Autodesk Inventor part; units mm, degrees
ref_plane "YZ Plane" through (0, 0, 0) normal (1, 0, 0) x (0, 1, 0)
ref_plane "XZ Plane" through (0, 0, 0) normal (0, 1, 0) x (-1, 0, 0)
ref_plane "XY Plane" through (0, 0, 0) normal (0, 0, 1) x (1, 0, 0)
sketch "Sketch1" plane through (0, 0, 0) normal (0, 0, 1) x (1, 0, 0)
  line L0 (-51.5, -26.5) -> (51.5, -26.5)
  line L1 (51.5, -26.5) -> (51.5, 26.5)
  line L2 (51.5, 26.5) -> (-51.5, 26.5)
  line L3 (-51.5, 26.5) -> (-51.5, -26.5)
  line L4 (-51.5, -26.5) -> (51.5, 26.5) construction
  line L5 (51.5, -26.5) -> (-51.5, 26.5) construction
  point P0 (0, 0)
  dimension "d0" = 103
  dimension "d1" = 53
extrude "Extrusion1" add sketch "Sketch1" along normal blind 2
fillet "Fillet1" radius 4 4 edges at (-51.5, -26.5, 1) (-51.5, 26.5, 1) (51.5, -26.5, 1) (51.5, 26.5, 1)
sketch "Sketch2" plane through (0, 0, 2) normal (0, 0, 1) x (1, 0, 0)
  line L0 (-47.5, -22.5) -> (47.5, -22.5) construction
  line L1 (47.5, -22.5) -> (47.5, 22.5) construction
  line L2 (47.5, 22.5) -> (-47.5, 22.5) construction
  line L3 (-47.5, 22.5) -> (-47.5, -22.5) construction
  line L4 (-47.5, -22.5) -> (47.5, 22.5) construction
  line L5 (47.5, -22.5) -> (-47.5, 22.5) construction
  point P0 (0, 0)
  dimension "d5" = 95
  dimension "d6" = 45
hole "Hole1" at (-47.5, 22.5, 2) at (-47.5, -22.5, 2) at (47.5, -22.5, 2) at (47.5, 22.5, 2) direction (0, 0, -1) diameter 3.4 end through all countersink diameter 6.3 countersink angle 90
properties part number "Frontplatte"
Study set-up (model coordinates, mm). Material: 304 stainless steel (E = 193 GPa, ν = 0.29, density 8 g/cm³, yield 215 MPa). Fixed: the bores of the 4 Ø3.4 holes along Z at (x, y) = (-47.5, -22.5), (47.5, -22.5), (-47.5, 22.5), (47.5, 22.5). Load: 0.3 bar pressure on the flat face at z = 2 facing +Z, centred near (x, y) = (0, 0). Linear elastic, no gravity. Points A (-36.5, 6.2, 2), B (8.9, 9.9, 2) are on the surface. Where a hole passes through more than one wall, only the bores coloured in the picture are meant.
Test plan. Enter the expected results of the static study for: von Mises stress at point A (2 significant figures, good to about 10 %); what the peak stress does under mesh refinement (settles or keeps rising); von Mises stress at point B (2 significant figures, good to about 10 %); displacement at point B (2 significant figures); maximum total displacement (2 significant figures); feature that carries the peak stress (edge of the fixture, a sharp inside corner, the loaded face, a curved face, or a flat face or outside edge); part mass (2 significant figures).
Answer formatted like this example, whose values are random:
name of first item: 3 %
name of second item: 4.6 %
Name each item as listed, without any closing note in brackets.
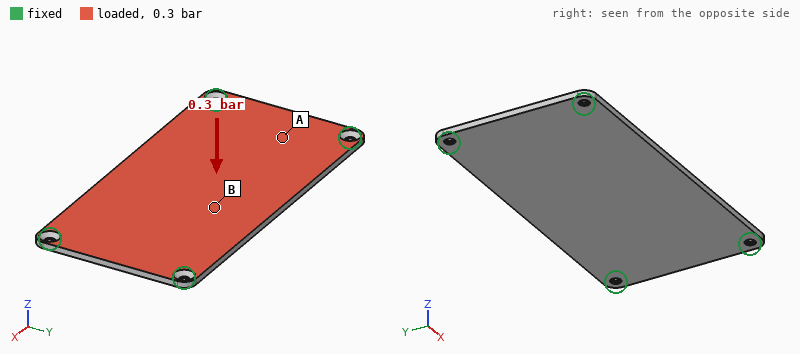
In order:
von Mises stress at point A: 9.1 MPa
what the peak stress does under mesh refinement: keeps rising
von Mises stress at point B: 22 MPa
displacement at point B: 80 µm
maximum total displacement: 87 µm
feature that carries the peak stress: edge of the fixture
part mass: 86 g
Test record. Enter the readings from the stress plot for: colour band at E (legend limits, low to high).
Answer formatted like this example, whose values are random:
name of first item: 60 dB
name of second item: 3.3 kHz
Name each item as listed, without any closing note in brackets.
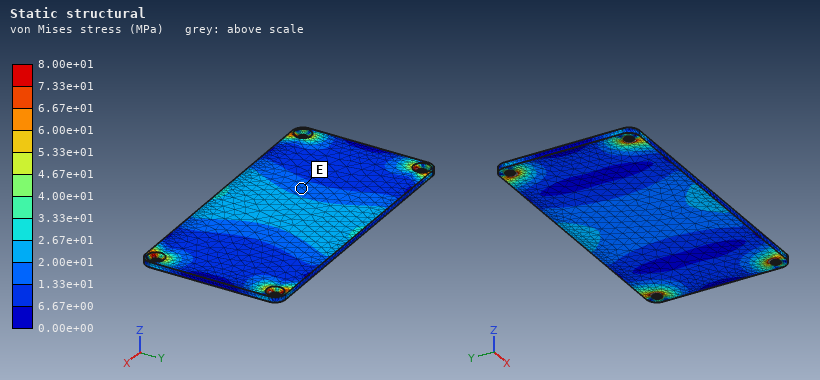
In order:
colour band at E: 1.33e+01 to 2.00e+01 MPa
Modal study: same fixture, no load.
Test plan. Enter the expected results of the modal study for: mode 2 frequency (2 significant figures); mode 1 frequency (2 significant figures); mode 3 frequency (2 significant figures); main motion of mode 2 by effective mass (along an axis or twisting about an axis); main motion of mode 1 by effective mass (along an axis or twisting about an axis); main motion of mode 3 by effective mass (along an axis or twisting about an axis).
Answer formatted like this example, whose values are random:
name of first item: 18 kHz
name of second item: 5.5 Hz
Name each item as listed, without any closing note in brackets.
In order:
mode 2 frequency: 1600 Hz
mode 1 frequency: 850 Hz
mode 3 frequency: 2400 Hz
main motion of mode 2 by effective mass: twisting about X
main motion of mode 1 by effective mass: along Z
main motion of mode 3 by effective mass: twisting about Y
